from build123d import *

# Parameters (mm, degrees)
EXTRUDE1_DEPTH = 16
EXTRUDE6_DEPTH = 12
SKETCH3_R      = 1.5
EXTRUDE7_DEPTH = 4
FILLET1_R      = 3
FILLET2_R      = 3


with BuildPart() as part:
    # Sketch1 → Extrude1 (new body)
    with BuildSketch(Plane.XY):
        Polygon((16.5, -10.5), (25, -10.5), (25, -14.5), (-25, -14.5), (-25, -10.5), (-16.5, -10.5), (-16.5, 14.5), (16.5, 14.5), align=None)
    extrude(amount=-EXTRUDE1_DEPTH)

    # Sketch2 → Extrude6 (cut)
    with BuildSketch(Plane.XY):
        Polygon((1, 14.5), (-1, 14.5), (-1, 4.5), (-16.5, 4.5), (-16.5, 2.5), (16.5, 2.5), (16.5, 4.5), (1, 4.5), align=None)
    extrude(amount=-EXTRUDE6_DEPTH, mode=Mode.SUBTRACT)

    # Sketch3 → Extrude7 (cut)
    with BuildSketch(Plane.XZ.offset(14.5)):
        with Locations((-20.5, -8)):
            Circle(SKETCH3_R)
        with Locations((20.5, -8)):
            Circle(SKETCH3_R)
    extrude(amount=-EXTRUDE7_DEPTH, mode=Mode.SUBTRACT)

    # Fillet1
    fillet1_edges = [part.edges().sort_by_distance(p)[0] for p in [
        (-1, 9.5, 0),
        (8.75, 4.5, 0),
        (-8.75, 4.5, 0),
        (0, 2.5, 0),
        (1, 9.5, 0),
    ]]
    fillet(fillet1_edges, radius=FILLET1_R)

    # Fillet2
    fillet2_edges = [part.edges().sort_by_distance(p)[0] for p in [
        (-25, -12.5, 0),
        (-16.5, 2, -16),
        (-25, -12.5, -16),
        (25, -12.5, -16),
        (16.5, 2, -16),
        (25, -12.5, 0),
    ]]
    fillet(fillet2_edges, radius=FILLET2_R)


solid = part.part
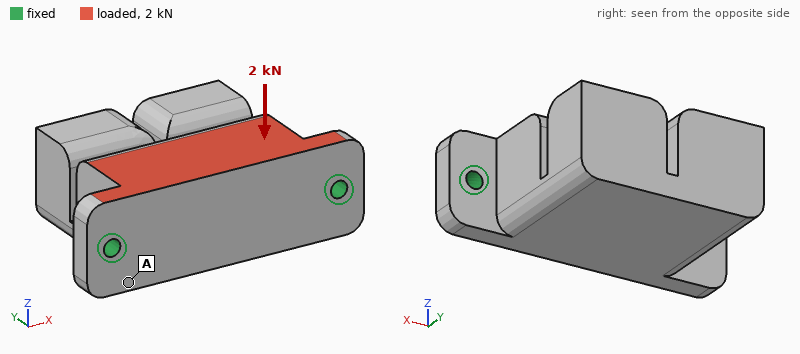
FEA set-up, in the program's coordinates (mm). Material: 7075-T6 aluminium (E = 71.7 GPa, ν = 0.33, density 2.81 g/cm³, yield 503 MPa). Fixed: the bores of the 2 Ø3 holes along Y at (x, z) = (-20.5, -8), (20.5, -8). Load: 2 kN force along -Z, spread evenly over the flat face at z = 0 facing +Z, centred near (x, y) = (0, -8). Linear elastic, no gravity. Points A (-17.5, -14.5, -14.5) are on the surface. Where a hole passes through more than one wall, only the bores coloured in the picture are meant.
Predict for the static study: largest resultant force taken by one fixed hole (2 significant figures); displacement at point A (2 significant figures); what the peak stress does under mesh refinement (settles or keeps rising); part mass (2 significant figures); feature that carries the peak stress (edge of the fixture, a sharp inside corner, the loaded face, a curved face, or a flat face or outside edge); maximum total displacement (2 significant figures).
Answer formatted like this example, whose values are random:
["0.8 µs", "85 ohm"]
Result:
["1.0 kN", "15 µm", "keeps rising", "42 g", "edge of the fixture", "93 µm"]
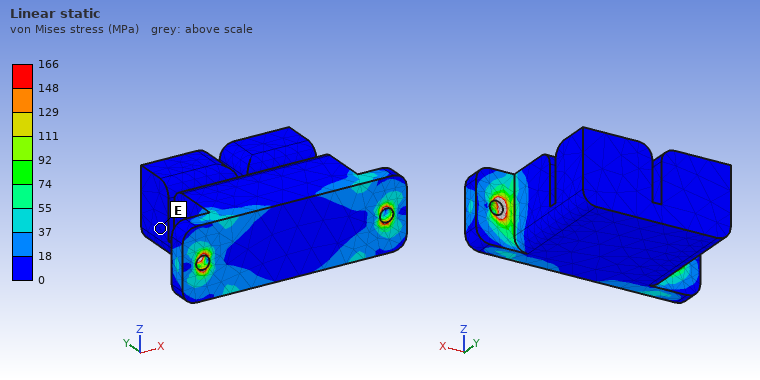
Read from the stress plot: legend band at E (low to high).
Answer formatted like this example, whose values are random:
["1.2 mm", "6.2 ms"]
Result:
["0 to 18 MPa"]
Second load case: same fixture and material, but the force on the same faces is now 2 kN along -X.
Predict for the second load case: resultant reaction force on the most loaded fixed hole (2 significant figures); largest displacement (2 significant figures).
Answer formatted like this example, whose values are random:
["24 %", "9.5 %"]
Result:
["1.1 kN", "7.9 µm"]
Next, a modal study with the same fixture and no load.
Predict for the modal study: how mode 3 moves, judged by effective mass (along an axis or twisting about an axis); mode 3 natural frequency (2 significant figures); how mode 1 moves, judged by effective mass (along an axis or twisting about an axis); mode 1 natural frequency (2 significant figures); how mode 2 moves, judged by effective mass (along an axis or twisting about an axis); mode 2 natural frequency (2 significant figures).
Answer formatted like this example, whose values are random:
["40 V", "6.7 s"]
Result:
["along X", "9000 Hz", "along Z", "2700 Hz", "along Y", "7700 Hz"]
